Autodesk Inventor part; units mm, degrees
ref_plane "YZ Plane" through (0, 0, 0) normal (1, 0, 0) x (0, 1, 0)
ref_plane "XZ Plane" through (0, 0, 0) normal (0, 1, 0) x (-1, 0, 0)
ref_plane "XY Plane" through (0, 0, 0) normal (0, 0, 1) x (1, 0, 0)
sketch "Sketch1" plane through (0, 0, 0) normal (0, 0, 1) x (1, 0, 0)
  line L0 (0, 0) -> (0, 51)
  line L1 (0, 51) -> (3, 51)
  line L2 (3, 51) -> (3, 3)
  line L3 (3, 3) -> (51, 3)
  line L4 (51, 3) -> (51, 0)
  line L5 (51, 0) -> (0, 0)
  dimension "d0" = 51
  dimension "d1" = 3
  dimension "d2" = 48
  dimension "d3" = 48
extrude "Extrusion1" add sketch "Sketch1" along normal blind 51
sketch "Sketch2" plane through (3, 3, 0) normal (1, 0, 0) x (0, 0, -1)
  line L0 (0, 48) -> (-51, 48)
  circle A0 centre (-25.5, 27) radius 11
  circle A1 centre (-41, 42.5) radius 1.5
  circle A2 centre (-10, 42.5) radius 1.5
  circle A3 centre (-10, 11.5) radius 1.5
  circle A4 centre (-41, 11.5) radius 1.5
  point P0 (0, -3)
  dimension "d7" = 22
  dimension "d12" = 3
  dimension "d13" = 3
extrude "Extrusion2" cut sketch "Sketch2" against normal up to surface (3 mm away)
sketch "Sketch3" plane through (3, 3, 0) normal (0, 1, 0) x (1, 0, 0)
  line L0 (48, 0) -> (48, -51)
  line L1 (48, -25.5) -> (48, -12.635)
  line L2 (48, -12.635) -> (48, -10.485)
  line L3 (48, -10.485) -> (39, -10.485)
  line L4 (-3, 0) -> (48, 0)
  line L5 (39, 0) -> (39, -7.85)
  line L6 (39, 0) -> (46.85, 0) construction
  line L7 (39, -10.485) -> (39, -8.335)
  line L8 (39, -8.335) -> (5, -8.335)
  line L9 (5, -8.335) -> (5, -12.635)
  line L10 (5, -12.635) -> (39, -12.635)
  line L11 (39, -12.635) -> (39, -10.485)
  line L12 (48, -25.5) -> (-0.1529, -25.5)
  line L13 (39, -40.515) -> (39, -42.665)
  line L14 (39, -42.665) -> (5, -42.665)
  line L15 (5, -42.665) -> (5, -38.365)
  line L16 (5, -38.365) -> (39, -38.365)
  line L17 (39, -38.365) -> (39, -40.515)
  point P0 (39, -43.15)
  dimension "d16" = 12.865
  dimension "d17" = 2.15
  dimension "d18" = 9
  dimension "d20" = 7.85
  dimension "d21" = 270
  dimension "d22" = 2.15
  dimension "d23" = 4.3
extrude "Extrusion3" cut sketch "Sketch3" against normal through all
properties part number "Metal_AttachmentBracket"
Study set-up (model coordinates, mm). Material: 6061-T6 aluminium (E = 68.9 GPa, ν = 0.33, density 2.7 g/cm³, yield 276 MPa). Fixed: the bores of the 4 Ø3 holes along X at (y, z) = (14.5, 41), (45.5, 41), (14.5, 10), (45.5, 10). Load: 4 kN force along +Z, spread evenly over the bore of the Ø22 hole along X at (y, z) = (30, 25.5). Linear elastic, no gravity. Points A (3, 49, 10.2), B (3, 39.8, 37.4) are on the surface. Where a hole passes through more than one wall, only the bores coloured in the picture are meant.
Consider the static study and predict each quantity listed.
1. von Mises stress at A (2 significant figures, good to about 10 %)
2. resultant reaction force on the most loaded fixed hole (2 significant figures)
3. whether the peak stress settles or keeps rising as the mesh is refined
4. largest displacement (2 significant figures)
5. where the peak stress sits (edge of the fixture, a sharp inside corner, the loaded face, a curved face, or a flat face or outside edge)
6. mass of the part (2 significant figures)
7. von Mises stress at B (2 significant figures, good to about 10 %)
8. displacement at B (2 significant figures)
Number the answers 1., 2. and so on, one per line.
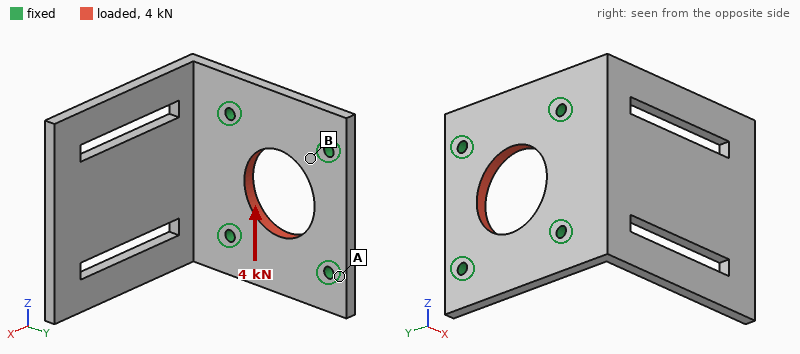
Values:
1. 10 MPa
2. 1.0 kN
3. keeps rising
4. 9.3 µm
5. edge of the fixture
6. 35 g
7. 23 MPa
8. 4.5 µm
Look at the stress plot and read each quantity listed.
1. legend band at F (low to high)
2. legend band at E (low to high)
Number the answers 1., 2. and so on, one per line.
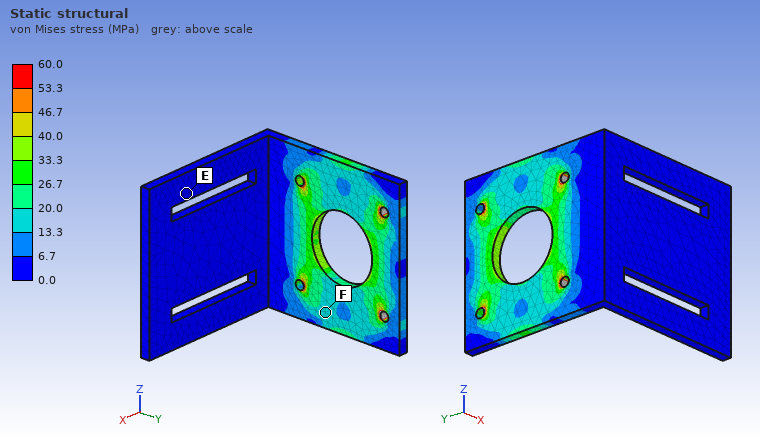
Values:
1. 13.3 to 20.0 MPa
2. 0.0 to 6.7 MPa
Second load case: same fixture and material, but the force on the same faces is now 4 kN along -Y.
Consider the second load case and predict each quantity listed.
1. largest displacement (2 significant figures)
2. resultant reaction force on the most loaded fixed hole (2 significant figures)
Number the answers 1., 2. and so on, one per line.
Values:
1. 13 µm
2. 1.0 kN
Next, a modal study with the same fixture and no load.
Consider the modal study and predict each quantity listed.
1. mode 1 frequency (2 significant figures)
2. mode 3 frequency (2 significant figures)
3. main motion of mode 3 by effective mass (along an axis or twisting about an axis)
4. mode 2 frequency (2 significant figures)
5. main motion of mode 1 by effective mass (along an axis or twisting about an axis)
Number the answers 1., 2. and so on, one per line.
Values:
1. 710 Hz
2. 2500 Hz
3. along Z
4. 1800 Hz
5. along Y
